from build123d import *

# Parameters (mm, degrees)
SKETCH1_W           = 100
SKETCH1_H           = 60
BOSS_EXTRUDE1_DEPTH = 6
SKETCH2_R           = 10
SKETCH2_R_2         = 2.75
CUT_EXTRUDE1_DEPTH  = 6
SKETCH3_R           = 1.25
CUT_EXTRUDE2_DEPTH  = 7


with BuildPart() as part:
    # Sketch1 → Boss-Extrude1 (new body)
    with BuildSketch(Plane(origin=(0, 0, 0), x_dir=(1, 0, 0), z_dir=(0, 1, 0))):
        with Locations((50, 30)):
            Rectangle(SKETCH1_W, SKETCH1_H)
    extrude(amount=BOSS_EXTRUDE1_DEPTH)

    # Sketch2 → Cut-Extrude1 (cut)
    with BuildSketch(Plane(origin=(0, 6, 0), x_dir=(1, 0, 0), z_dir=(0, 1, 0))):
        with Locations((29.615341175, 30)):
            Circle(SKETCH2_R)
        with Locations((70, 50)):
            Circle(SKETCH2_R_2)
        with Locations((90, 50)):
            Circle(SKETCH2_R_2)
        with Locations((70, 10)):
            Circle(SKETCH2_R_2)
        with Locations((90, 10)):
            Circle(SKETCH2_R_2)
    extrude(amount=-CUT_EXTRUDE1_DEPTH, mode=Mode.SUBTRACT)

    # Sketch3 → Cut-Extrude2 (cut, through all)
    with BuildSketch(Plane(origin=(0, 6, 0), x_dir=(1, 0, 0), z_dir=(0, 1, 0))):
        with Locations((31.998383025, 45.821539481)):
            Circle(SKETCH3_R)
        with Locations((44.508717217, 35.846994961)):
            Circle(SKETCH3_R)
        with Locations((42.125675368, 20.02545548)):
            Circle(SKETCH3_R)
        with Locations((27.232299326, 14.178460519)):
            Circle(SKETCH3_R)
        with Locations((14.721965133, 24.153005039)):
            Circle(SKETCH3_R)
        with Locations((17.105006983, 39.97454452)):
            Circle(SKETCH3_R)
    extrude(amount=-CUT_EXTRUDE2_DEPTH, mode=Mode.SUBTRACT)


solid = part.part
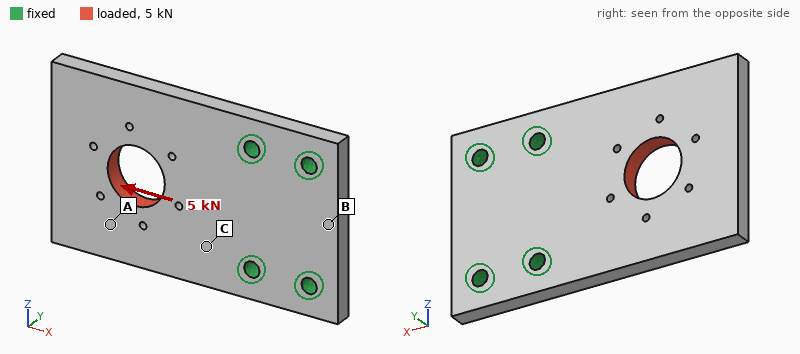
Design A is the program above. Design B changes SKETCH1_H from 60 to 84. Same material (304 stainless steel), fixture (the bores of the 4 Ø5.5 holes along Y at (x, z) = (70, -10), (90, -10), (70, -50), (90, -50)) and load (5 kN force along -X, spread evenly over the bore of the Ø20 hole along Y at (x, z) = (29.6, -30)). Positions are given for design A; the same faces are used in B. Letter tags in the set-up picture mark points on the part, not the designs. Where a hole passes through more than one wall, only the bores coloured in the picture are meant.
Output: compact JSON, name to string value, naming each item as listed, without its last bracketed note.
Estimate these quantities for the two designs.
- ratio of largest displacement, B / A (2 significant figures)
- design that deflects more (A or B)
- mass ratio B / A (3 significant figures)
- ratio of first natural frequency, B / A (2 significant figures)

{"ratio of largest displacement, B / A": "0.92", "design that deflects more": "A", "mass ratio B / A": "1.43", "ratio of first natural frequency, B / A": "0.99"}
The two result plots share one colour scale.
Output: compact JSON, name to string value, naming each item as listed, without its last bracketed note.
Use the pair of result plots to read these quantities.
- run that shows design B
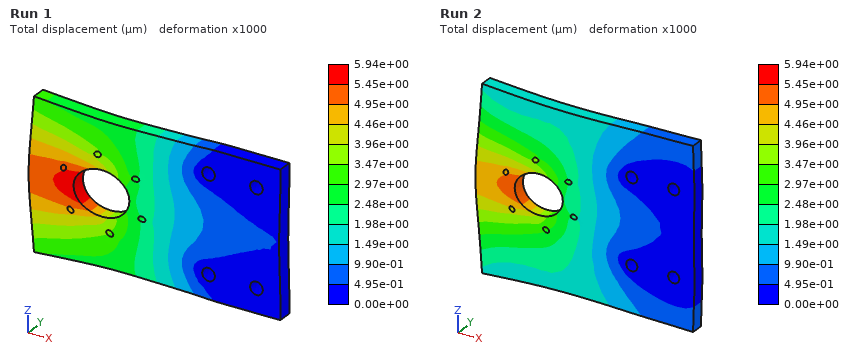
{"run that shows design B": "Run 2"}
